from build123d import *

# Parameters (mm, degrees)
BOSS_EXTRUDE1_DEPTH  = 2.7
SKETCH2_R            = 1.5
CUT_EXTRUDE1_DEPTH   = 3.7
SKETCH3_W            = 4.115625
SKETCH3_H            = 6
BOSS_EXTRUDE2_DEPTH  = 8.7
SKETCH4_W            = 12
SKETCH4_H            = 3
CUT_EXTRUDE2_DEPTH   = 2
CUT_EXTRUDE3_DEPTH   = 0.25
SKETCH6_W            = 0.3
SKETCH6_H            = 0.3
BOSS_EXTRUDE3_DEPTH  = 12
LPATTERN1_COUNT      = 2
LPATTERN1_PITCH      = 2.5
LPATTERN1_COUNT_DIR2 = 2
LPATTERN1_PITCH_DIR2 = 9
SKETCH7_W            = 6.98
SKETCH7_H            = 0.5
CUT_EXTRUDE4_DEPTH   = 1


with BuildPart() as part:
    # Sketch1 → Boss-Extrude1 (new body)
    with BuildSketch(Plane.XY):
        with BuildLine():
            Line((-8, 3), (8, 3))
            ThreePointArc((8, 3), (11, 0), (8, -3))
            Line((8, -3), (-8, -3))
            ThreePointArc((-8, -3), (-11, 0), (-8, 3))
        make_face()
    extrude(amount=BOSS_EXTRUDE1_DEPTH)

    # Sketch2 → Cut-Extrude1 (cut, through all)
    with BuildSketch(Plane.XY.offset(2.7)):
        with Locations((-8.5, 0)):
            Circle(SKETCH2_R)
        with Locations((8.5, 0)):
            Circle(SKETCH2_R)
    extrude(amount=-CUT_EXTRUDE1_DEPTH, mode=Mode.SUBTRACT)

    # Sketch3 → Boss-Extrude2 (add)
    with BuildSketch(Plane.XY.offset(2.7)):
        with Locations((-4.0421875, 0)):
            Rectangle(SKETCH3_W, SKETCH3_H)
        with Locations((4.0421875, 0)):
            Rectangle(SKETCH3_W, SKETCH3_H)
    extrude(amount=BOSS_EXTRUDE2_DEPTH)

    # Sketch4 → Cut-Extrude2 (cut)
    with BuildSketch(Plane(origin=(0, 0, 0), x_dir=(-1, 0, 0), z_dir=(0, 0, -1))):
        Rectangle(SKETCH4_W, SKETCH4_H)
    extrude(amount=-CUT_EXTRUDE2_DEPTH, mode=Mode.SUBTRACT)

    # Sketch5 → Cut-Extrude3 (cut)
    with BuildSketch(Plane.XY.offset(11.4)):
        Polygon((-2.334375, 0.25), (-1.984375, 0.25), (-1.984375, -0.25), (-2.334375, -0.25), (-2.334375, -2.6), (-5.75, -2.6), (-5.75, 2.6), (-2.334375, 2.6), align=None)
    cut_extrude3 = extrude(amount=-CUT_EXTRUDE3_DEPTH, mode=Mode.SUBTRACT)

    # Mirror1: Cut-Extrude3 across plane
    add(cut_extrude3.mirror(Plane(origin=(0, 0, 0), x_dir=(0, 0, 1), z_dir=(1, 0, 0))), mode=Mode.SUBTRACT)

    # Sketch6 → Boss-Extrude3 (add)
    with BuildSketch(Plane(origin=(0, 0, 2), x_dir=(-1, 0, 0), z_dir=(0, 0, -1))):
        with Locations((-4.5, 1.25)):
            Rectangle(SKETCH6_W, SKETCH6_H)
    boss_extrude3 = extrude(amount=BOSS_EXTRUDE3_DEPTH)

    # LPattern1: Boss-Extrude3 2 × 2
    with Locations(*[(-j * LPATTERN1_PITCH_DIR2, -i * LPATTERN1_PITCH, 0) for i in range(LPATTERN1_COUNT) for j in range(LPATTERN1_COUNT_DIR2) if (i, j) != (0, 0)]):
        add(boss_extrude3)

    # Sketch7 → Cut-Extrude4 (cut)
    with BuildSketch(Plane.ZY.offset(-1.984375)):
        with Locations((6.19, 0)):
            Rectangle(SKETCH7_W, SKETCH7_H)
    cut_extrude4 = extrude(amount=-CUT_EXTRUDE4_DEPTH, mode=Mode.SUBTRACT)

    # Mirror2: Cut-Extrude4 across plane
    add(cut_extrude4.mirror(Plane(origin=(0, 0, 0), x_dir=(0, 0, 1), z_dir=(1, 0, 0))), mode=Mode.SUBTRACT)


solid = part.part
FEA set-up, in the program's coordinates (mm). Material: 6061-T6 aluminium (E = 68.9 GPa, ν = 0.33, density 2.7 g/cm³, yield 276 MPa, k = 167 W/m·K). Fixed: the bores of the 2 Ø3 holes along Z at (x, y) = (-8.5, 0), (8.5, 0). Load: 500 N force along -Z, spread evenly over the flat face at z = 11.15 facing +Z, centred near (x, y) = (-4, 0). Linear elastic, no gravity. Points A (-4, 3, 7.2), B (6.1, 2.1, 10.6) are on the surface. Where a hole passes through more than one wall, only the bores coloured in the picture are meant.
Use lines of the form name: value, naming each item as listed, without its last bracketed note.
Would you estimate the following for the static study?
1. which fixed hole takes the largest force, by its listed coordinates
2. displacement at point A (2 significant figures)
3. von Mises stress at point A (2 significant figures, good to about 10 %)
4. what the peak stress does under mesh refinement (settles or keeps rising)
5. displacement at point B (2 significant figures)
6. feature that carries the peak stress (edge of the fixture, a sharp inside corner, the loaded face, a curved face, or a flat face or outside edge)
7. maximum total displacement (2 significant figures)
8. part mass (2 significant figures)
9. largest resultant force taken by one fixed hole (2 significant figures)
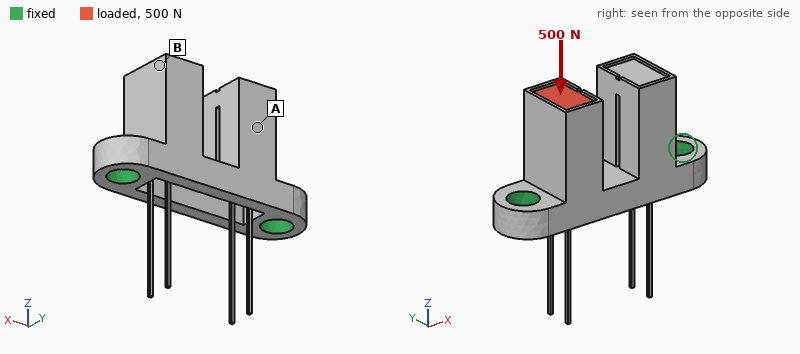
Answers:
which fixed hole takes the largest force, by its listed coordinates: (-8.5, 0)
displacement at point A: 19 µm
von Mises stress at point A: 20 MPa
what the peak stress does under mesh refinement: keeps rising
displacement at point B: 18 µm
feature that carries the peak stress: edge of the fixture
maximum total displacement: 37 µm
part mass: 1.7 g
largest resultant force taken by one fixed hole: 410 N
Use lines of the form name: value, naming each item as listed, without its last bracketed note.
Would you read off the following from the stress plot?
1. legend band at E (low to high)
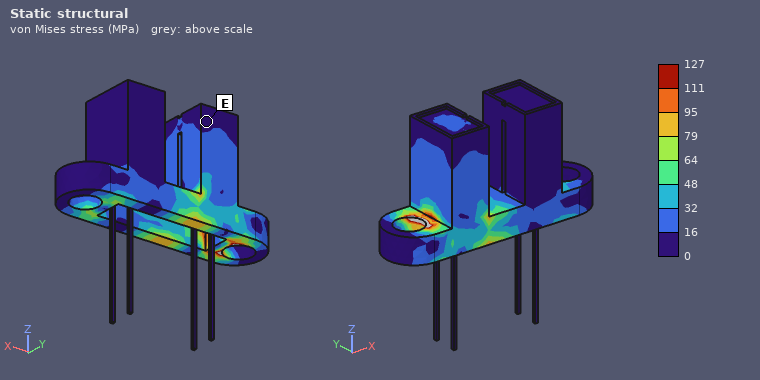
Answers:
legend band at E: 0 to 16 MPa
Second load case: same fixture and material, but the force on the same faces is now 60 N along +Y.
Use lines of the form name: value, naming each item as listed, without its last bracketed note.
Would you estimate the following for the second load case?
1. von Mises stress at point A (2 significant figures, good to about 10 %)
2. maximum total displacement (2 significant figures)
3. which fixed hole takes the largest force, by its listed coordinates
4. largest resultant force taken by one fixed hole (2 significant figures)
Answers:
von Mises stress at point A: 9.9 MPa
maximum total displacement: 18 µm
which fixed hole takes the largest force, by its listed coordinates: (-8.5, 0)
largest resultant force taken by one fixed hole: 49 N
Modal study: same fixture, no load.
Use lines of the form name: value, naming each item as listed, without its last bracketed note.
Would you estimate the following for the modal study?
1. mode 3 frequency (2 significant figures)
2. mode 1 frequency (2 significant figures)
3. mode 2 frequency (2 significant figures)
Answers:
mode 3 frequency: 1700 Hz
mode 1 frequency: 1700 Hz
mode 2 frequency: 1700 Hz
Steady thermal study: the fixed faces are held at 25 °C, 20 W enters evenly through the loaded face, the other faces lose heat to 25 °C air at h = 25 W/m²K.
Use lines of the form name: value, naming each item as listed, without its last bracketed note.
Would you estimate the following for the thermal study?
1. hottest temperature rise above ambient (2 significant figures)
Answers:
hottest temperature rise above ambient: 65 K
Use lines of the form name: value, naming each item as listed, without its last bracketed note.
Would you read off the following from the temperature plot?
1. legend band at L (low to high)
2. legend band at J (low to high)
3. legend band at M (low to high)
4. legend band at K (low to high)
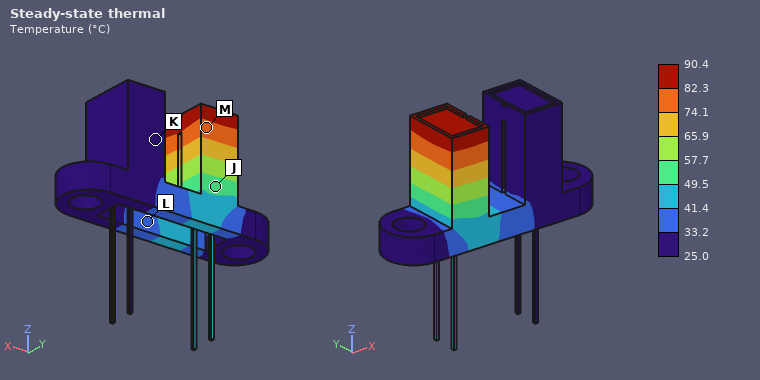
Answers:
legend band at L: 33.2 to 41.4 °C
legend band at J: 49.5 to 57.7 °C
legend band at M: 74.1 to 82.3 °C
legend band at K: 25.0 to 33.2 °C
